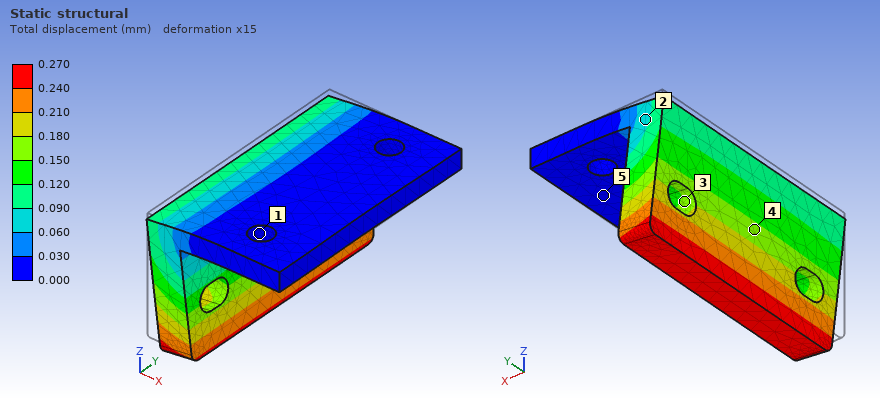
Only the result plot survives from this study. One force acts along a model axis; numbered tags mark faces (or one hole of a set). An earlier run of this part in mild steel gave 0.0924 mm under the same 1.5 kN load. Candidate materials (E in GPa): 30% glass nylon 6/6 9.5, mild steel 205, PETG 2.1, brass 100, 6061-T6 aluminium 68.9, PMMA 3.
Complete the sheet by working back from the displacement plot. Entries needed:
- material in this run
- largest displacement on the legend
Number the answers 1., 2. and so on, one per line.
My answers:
1. 6061-T6 aluminium
2. 0.270 mm
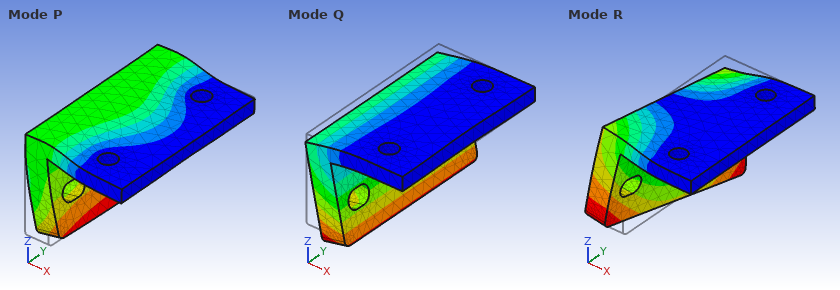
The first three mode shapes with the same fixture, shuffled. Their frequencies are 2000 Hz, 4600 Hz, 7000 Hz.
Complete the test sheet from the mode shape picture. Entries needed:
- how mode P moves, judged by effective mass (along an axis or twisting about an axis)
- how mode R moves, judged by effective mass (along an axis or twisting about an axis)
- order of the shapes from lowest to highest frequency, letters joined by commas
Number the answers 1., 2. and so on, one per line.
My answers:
1. along Z
2. along Y
3. Q, R, P
